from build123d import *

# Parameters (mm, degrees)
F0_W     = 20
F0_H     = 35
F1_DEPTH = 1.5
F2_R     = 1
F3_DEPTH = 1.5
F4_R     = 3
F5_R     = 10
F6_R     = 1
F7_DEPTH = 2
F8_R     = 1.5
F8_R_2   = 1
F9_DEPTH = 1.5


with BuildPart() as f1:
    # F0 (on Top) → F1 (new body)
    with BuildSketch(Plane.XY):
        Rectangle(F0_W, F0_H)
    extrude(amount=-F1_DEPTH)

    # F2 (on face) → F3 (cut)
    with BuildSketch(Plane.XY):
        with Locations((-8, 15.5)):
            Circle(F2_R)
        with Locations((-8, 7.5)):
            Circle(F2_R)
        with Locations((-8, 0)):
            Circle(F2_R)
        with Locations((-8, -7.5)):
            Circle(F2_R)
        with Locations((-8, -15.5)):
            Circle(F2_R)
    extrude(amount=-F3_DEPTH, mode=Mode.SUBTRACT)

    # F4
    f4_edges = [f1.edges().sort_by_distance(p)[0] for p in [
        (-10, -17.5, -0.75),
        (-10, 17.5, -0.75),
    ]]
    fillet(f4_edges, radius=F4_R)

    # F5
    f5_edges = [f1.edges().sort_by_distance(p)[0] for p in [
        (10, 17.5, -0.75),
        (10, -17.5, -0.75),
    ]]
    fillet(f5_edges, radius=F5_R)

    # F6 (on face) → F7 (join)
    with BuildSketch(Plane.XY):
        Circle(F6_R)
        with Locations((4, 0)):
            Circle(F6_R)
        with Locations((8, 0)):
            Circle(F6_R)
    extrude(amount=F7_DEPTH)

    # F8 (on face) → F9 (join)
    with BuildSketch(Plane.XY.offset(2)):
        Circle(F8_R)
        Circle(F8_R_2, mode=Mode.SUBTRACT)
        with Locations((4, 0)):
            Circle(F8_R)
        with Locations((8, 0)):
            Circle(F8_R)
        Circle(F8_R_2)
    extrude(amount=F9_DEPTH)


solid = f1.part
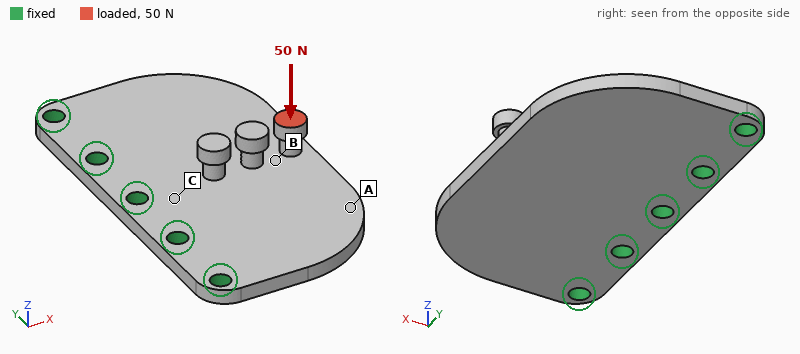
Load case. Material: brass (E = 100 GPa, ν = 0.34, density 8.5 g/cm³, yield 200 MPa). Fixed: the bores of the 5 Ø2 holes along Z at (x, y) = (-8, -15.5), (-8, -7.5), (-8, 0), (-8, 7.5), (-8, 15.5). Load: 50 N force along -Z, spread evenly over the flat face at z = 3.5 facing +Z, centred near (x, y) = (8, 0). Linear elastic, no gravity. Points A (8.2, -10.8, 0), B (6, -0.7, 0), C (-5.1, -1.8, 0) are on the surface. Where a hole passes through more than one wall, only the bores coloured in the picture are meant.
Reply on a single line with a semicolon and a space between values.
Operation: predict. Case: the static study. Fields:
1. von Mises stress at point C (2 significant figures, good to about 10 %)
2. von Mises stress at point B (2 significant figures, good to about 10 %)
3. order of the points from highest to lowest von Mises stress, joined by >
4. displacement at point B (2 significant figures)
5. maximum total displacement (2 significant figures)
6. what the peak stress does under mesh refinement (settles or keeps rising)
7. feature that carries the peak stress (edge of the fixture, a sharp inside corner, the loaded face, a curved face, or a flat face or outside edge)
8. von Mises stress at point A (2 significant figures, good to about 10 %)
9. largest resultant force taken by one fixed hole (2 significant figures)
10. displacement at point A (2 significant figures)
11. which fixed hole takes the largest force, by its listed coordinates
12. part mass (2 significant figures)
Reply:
54 MPa; 29 MPa; C > B > A; 62 µm; 93 µm; keeps rising; edge of the fixture; 14 MPa; 21 N; 60 µm; (-8, 0); 8.6 g
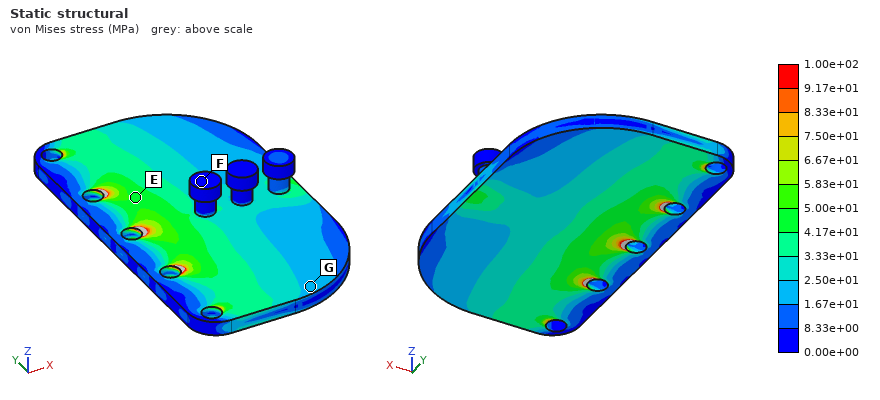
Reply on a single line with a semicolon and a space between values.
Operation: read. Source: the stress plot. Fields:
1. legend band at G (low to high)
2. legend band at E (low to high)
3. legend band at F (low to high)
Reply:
1.67e+01 to 2.50e+01 MPa; 4.17e+01 to 5.00e+01 MPa; 0.00e+00 to 8.33e+00 MPa
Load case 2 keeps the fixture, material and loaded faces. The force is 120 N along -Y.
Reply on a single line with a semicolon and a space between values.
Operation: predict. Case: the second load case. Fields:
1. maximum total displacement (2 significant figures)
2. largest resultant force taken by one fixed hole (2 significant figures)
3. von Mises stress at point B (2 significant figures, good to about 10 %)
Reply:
72 µm; 54 N; 100 MPa
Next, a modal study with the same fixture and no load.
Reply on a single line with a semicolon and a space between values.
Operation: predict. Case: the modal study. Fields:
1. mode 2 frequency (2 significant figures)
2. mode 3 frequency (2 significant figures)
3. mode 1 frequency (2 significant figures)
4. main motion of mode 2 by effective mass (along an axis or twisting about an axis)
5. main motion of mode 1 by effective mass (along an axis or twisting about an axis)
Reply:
5200 Hz; 9400 Hz; 2800 Hz; twisting about X; along Z
